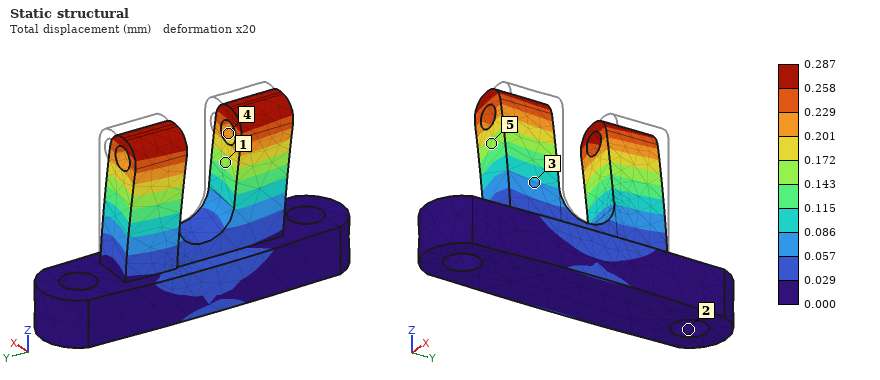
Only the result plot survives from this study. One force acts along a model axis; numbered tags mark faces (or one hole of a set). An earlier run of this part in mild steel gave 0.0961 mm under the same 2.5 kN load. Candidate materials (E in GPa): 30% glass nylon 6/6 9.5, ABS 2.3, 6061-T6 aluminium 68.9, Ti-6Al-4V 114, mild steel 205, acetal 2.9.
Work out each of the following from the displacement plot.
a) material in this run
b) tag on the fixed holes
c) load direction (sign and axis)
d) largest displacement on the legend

6061-T6 aluminium
2
-X
0.287 mm
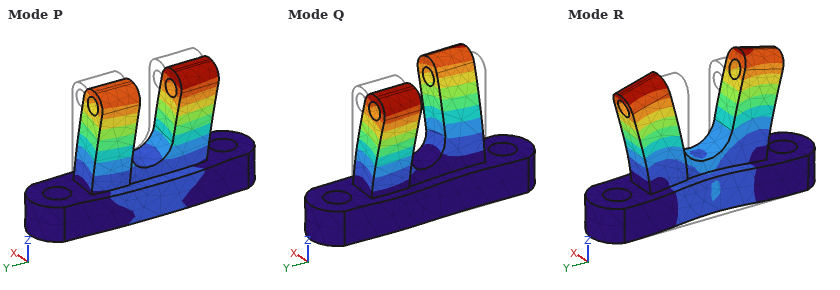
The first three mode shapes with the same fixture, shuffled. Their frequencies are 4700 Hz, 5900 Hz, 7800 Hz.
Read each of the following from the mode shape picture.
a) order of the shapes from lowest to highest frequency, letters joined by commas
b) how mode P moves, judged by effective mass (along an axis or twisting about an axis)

P, Q, R
along X
